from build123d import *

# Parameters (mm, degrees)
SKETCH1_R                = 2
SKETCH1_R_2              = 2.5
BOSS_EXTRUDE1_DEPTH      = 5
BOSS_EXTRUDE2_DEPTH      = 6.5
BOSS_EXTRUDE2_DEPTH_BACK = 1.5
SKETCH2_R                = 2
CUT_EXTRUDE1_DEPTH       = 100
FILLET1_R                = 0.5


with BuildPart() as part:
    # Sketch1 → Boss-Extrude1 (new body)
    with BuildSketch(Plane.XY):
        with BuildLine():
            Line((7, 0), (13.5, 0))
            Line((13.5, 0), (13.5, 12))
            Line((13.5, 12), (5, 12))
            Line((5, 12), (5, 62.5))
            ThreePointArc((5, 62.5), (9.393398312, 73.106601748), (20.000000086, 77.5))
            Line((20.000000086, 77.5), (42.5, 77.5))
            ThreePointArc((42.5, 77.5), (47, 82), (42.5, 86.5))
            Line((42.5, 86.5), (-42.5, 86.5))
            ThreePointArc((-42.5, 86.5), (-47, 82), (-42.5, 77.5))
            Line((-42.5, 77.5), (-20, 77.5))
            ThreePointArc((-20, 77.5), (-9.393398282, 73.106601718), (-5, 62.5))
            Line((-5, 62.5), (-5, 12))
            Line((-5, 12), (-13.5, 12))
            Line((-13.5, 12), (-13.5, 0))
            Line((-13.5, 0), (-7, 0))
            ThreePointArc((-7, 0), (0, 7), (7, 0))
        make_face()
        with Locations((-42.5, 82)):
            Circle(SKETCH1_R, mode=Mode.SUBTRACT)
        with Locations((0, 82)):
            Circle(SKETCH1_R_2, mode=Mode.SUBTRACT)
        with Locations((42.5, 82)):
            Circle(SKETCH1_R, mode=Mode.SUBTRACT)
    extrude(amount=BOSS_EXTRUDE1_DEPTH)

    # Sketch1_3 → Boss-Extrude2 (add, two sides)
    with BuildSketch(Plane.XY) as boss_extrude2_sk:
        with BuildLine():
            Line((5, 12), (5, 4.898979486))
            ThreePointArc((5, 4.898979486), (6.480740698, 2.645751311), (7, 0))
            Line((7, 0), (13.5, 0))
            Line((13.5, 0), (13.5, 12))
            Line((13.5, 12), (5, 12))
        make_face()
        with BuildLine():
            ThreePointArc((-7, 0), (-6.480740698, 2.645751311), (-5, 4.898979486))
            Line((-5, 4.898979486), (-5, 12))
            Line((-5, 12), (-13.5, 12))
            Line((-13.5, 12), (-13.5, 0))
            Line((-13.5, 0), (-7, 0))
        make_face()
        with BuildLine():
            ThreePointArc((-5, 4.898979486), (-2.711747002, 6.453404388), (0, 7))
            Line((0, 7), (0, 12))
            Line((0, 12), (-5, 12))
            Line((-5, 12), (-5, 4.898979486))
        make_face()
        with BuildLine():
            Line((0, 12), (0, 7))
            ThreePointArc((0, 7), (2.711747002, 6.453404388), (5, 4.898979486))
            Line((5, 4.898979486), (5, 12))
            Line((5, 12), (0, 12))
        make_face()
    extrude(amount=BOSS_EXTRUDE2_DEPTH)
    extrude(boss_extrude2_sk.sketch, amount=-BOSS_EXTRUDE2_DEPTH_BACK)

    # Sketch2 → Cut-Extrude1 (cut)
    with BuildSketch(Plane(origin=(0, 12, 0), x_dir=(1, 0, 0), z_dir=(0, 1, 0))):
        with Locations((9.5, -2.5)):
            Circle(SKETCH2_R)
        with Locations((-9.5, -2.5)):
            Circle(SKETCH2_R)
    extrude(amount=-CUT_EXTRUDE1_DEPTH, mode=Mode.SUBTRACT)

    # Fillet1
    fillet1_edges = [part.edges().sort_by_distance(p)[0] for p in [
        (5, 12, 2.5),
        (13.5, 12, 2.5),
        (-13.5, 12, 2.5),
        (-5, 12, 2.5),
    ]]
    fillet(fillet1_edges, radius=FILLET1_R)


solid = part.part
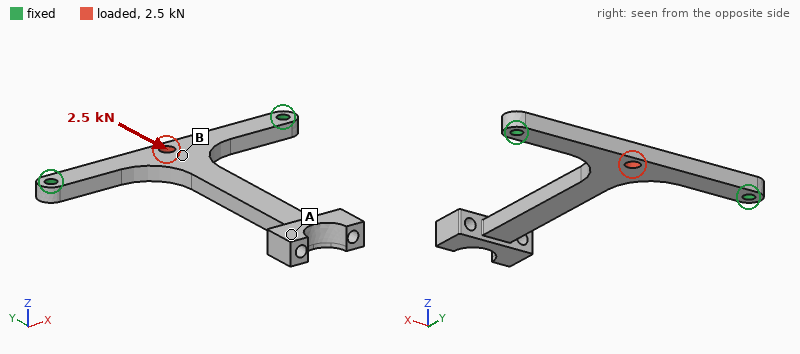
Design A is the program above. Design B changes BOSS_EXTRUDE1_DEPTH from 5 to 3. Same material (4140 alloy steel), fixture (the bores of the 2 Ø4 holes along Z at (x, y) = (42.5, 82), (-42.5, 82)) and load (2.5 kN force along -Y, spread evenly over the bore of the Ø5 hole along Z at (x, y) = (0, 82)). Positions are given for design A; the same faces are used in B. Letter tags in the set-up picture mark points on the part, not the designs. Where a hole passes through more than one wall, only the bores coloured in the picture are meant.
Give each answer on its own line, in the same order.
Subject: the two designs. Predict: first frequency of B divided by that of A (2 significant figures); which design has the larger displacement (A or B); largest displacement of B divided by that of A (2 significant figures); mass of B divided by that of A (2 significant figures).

0.52
B
1.7
0.67
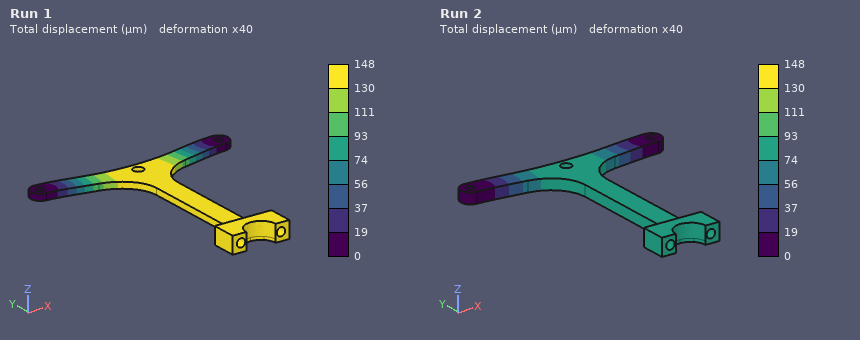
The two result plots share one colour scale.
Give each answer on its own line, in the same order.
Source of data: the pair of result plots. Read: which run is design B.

Run 1
